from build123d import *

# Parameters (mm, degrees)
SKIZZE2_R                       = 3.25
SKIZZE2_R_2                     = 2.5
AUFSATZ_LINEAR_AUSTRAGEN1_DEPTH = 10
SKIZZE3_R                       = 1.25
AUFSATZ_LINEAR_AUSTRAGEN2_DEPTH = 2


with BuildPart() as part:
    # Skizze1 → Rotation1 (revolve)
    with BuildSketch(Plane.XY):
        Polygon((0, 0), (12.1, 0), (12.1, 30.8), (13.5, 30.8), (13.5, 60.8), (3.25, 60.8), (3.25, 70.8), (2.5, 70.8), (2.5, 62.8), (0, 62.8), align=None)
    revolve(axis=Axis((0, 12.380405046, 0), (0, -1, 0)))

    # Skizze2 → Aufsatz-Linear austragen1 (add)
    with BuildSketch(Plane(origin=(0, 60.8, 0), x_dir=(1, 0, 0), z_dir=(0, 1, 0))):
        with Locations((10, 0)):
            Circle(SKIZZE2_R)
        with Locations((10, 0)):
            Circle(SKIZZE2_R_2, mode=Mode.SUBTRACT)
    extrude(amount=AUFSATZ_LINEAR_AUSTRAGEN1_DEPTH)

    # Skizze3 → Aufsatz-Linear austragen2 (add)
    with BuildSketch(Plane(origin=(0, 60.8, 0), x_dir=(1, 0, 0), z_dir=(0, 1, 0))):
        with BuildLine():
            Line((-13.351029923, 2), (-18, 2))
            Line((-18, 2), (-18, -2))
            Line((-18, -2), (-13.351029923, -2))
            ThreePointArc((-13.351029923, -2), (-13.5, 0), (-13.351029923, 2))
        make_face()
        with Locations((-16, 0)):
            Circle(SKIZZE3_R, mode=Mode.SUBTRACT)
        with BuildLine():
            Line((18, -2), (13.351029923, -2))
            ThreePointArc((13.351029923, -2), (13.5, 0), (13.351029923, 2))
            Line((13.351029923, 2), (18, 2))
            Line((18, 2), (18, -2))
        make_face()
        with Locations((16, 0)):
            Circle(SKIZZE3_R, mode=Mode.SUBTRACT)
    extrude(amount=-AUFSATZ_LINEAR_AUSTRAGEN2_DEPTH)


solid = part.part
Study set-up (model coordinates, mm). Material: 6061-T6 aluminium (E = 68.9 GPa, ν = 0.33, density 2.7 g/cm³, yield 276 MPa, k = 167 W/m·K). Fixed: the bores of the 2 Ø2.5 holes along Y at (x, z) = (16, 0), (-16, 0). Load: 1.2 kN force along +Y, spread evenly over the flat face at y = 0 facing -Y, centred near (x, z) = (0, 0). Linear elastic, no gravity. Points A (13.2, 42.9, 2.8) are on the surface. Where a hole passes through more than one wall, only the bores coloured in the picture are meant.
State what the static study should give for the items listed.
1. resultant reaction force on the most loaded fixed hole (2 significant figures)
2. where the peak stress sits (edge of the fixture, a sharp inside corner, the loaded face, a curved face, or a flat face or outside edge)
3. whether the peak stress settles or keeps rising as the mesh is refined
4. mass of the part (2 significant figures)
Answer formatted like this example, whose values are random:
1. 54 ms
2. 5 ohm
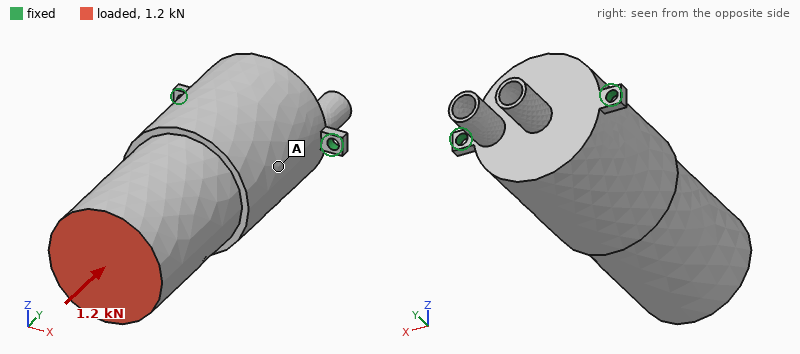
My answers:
1. 660 N
2. edge of the fixture
3. keeps rising
4. 86 g
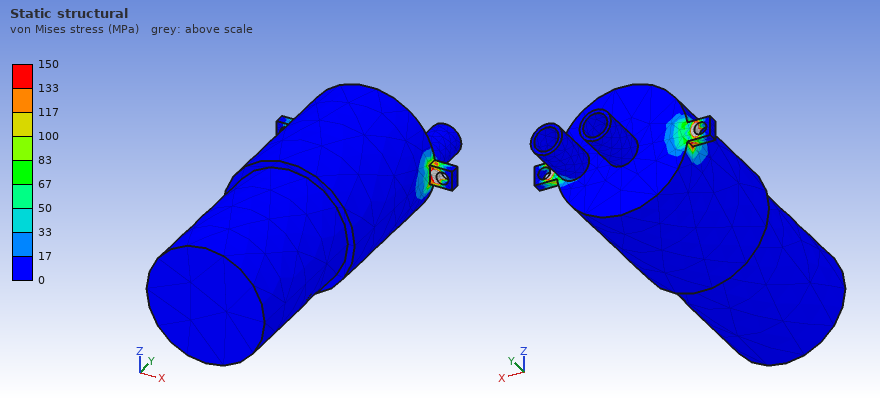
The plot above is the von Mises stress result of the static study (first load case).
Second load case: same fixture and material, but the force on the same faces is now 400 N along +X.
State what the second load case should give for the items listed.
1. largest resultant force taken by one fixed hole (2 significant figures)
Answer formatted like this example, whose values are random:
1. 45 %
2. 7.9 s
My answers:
1. 890 N
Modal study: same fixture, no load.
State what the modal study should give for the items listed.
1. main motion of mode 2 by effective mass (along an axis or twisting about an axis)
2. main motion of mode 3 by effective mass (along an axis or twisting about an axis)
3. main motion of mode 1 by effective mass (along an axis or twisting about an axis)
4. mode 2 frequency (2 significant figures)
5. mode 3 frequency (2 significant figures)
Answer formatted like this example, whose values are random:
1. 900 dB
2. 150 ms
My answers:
1. along X
2. along Y
3. along Z
4. 2100 Hz
5. 5100 Hz
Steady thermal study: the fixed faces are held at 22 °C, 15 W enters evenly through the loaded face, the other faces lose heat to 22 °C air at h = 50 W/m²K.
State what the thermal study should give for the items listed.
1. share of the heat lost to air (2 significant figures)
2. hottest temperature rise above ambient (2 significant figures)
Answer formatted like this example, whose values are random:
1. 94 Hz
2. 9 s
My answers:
1. 31 %
2. 21 K
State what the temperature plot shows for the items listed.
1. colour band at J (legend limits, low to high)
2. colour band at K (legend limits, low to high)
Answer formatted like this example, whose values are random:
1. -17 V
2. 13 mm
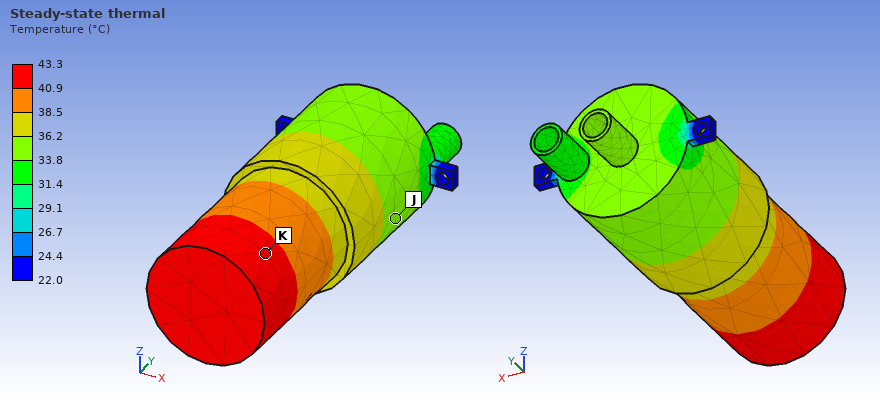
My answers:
1. 33.8 to 36.2 °C
2. 40.9 to 43.3 °C
